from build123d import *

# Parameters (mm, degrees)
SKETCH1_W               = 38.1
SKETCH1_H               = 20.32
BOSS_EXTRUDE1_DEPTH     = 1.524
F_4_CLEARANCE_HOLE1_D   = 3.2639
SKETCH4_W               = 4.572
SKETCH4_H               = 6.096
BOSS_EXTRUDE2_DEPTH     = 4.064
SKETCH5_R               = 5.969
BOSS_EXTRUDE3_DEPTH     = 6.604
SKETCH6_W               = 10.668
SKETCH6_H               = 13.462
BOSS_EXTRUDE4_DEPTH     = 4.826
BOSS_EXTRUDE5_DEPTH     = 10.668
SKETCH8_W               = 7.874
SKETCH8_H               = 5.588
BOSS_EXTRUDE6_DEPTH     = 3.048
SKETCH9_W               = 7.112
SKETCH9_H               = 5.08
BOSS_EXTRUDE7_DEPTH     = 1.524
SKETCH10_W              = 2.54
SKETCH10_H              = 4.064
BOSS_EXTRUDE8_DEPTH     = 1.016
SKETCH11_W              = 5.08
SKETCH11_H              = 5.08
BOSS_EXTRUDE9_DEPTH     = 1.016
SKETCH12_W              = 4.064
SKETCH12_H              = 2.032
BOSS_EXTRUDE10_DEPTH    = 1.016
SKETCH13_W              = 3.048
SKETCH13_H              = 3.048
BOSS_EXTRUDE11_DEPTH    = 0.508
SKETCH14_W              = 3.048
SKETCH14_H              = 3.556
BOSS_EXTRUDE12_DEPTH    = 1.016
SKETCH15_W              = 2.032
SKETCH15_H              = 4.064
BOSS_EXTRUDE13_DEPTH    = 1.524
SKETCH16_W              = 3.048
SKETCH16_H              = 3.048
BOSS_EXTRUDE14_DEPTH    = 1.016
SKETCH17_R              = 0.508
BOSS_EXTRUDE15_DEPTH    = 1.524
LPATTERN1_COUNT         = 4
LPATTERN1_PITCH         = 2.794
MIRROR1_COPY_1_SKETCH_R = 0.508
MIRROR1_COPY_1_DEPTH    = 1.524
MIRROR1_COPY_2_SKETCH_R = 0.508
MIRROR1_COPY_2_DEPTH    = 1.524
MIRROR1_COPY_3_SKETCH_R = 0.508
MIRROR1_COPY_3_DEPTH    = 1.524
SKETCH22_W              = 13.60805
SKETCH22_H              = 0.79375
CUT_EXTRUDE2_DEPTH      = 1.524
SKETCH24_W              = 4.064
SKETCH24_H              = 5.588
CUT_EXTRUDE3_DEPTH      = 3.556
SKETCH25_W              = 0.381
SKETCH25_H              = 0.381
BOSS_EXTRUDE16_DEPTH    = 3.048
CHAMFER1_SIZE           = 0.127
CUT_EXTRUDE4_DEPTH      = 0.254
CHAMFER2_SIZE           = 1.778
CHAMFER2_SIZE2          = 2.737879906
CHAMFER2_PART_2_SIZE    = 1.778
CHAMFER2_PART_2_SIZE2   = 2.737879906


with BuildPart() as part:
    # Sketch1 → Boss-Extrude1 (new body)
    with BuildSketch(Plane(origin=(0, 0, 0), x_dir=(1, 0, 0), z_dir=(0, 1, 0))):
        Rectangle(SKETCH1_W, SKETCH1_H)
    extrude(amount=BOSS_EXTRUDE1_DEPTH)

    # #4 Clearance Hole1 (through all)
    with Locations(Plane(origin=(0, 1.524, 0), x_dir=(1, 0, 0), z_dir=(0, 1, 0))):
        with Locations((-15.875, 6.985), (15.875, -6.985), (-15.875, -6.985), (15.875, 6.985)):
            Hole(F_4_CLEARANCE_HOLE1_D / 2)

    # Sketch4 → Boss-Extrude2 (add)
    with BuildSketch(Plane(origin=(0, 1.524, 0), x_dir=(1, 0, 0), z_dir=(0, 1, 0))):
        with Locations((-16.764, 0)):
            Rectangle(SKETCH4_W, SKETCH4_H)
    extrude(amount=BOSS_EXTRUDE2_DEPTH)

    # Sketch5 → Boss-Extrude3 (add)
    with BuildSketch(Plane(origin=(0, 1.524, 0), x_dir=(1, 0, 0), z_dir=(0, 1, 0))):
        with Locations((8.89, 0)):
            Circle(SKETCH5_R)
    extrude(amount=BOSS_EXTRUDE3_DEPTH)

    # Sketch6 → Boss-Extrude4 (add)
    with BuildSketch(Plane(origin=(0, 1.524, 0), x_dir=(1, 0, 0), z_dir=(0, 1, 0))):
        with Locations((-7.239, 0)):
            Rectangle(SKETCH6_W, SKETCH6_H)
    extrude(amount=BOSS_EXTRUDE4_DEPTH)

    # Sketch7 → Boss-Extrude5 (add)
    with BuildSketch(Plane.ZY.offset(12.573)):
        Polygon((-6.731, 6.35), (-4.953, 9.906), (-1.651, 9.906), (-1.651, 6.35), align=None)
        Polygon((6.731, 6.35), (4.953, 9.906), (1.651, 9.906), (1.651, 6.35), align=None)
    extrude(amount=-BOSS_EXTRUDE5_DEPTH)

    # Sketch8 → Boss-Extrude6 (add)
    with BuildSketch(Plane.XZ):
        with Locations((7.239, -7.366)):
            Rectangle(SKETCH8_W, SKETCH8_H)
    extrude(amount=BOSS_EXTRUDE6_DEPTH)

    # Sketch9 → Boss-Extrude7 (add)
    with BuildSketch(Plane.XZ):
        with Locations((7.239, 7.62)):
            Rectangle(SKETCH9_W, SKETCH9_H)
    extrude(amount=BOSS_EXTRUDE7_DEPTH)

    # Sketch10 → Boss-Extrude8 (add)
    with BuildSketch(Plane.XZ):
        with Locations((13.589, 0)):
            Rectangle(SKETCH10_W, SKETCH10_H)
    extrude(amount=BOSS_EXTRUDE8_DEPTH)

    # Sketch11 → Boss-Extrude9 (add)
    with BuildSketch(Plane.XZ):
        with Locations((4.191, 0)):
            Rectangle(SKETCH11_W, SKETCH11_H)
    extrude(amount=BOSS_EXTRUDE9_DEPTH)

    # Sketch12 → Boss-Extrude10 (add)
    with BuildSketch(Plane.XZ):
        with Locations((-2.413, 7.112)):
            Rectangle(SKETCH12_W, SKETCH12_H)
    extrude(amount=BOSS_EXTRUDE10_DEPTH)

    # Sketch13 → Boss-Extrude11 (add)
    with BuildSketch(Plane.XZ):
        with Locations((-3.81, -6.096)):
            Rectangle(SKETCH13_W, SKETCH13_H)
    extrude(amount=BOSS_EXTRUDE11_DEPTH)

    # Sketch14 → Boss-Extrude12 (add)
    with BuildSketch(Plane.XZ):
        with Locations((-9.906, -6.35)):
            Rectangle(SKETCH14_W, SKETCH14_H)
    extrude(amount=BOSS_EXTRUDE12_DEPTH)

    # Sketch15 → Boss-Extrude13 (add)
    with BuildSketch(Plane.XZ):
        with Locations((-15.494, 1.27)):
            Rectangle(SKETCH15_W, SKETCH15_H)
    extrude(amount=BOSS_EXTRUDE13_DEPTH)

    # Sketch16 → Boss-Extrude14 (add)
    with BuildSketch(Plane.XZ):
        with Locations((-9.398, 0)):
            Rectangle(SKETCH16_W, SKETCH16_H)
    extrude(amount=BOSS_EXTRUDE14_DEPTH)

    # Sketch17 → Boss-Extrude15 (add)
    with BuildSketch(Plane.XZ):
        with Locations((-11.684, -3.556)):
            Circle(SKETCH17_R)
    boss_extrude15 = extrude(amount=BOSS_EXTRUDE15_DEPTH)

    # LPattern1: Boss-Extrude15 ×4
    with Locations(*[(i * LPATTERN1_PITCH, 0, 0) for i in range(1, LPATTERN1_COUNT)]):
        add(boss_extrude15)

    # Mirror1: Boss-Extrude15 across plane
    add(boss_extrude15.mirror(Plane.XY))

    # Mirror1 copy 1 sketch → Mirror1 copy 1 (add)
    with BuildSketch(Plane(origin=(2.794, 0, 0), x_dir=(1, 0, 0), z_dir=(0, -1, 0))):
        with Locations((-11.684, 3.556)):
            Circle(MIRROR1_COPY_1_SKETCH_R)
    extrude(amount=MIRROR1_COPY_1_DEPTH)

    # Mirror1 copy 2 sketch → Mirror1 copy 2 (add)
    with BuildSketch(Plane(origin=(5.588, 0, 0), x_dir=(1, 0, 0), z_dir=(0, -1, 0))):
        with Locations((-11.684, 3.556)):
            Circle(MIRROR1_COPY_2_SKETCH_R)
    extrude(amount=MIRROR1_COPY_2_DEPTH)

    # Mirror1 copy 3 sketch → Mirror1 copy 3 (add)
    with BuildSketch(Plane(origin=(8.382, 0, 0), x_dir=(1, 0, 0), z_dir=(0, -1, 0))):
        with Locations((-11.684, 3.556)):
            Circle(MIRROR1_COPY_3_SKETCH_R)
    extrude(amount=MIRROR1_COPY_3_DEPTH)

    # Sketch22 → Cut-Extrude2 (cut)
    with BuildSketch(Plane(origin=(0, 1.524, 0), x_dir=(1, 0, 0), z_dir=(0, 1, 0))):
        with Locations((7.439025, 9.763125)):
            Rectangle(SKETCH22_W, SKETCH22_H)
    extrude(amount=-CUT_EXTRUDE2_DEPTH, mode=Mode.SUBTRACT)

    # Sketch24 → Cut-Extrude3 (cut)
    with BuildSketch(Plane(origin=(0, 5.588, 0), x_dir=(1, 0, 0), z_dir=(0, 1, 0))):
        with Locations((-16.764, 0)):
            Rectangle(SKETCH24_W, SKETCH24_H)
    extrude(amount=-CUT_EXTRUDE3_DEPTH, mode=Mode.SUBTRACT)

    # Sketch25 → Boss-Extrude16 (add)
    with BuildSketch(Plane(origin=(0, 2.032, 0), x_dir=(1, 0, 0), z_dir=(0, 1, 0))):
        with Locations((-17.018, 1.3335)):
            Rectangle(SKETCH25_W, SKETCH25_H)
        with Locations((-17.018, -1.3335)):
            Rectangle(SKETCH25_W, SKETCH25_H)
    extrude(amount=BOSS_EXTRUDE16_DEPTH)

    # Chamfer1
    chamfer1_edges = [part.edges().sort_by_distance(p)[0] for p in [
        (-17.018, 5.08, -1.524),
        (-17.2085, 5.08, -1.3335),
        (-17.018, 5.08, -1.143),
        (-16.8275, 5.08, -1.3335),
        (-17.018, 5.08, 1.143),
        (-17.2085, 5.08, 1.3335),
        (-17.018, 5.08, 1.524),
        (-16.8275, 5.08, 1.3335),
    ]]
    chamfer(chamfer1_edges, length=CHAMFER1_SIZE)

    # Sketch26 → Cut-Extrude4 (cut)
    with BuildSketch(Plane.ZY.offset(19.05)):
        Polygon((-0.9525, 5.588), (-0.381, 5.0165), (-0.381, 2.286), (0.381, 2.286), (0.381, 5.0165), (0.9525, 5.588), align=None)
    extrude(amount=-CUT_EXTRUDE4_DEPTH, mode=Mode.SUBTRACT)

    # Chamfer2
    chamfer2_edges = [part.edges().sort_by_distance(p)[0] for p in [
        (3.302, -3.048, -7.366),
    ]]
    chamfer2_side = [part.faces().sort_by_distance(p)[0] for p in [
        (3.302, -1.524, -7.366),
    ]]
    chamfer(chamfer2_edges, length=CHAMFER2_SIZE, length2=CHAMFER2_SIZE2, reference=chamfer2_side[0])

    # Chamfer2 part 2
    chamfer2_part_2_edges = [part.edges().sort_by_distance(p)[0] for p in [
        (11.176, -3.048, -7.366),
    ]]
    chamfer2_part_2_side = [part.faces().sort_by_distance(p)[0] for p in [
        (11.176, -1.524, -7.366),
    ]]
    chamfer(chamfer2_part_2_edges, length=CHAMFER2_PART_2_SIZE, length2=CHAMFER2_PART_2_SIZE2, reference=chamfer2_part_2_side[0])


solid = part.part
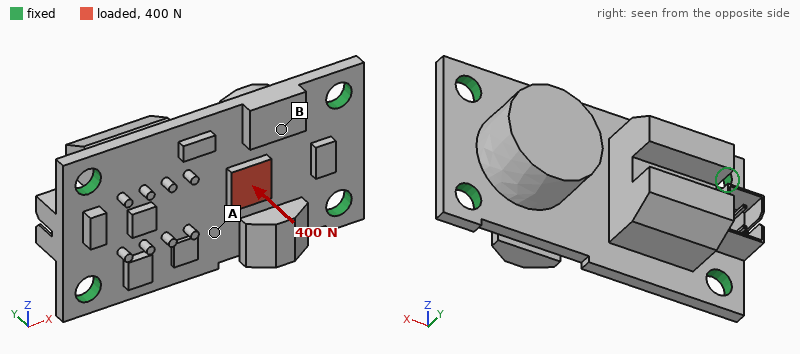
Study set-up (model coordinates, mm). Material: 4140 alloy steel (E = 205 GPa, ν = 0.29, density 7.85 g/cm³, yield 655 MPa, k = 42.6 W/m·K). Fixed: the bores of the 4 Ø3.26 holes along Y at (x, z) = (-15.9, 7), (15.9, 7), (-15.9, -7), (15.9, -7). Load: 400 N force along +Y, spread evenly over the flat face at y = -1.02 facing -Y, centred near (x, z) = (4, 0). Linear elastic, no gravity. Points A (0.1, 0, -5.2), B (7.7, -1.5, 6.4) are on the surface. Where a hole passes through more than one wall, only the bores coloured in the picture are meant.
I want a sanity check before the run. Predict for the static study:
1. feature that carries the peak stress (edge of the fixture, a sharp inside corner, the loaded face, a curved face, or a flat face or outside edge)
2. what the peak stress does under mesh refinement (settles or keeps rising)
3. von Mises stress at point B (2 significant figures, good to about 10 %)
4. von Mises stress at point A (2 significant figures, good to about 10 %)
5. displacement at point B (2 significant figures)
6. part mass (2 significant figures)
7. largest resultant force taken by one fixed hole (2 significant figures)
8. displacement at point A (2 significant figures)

edge of the fixture
keeps rising
17 MPa
98 MPa
16 µm
25 g
150 N
27 µm
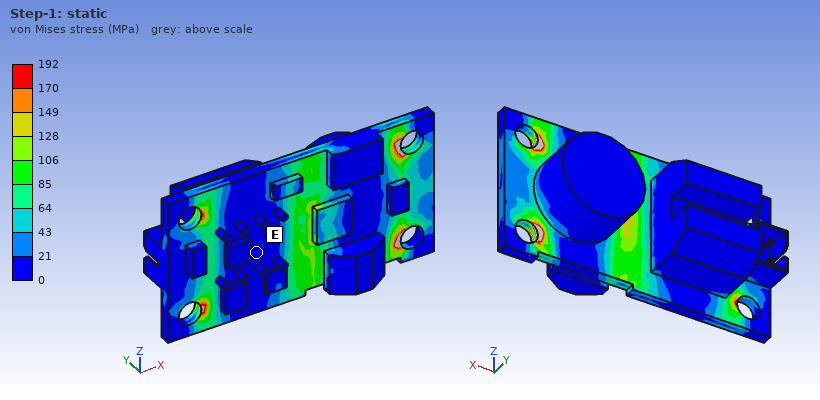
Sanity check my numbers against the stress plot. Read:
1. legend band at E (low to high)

0 to 21 MPa
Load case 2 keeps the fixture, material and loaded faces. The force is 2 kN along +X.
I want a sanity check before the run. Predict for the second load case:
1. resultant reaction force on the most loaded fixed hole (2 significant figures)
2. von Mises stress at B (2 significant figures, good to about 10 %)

620 N
16 MPa
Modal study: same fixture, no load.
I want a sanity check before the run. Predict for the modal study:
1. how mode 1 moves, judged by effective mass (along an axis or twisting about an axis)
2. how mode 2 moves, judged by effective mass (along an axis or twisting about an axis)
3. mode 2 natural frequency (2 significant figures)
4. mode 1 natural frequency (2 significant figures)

along Y
along Z
17 kHz
5600 Hz
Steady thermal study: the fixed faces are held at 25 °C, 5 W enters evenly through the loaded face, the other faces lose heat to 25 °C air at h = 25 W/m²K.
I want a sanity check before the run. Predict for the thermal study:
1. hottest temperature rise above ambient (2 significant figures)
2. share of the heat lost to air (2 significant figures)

27 K
10 %
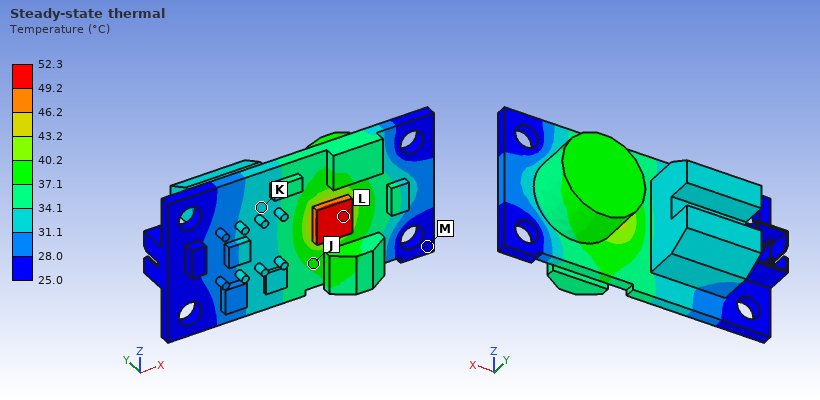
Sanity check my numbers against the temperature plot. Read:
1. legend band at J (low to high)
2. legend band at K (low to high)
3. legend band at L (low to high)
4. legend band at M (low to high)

37.1 to 40.2 °C
31.1 to 34.1 °C
49.2 to 52.3 °C
25.0 to 28.0 °C
